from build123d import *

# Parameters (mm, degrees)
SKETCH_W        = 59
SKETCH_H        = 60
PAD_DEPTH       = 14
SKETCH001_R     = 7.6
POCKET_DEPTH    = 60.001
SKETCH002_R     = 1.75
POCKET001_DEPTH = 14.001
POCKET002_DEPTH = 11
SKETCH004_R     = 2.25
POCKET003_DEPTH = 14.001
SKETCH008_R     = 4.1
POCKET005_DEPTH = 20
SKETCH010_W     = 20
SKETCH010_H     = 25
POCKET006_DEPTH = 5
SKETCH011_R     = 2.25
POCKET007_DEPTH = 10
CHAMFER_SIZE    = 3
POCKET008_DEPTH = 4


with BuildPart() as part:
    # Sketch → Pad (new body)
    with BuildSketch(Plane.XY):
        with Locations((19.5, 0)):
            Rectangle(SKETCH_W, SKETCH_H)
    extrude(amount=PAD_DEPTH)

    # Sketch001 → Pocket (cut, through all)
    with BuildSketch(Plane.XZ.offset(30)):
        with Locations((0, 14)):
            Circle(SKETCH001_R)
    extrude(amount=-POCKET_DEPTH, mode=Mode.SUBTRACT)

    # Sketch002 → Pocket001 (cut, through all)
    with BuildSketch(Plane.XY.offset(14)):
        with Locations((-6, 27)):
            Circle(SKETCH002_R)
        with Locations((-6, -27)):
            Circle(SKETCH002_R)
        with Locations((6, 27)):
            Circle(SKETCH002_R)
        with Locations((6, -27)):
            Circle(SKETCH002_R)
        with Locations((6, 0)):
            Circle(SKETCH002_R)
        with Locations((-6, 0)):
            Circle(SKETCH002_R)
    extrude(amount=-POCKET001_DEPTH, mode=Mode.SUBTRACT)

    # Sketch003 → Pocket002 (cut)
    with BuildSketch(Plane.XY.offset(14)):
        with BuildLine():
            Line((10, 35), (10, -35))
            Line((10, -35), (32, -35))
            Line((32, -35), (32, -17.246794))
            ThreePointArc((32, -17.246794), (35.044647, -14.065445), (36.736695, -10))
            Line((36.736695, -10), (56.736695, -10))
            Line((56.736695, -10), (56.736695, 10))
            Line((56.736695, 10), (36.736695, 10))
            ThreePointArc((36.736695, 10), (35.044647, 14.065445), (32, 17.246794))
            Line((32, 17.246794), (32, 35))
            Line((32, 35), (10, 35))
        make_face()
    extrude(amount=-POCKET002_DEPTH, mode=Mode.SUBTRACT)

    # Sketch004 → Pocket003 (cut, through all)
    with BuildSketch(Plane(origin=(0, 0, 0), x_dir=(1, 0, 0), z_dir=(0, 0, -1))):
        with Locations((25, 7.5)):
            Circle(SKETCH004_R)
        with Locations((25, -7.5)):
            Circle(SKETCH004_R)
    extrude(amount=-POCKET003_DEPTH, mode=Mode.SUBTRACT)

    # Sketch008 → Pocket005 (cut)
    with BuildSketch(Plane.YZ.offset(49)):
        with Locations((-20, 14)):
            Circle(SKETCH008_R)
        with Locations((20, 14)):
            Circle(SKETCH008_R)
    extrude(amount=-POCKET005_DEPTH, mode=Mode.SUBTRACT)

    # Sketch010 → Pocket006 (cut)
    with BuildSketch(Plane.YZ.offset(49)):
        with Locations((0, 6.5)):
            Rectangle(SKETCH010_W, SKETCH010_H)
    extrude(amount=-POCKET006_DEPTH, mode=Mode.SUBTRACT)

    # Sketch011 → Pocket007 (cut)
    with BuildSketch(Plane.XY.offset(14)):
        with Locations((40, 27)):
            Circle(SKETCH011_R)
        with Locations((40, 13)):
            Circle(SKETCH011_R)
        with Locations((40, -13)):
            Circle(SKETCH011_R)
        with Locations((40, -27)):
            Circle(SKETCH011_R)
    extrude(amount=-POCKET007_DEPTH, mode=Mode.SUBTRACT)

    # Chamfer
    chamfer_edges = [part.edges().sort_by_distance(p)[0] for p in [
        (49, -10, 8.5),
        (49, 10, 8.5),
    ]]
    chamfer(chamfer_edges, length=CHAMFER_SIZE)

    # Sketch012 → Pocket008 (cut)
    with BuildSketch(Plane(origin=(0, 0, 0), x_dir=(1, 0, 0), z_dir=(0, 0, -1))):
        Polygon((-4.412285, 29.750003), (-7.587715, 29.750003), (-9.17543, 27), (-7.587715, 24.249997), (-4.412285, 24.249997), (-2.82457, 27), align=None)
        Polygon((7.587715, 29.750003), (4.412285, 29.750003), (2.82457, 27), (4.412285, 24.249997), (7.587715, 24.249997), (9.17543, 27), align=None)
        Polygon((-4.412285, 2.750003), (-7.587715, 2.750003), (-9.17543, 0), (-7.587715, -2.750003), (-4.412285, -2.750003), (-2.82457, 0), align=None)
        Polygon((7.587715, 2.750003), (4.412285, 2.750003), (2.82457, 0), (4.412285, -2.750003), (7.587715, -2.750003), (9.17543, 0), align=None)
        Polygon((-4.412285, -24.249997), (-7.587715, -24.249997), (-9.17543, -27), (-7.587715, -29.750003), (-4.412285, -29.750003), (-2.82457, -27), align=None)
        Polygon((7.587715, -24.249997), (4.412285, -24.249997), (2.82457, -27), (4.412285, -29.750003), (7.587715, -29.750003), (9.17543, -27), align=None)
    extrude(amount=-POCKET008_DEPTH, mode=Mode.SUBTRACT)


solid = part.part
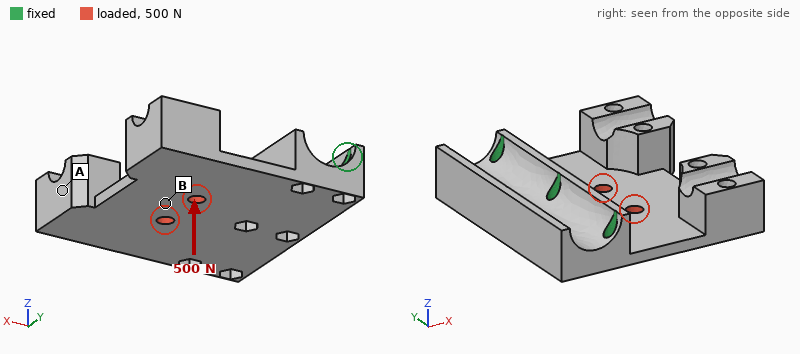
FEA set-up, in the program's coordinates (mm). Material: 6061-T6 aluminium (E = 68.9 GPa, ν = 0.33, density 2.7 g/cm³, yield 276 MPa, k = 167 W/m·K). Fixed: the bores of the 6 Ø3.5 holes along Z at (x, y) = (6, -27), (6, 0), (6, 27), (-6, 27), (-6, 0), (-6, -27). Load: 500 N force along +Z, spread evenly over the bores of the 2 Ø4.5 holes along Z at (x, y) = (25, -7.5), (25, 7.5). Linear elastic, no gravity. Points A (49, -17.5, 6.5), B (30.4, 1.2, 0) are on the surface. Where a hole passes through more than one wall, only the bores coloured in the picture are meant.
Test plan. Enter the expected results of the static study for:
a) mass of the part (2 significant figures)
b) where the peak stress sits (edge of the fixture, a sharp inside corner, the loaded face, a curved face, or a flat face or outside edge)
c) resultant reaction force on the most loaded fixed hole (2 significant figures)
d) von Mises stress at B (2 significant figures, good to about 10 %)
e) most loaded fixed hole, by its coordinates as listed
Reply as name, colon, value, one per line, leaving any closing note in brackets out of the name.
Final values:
mass of the part: 60 g
where the peak stress sits: a flat face or outside edge
resultant reaction force on the most loaded fixed hole: 690 N
von Mises stress at B: 14 MPa
most loaded fixed hole, by its coordinates as listed: (6, 0)
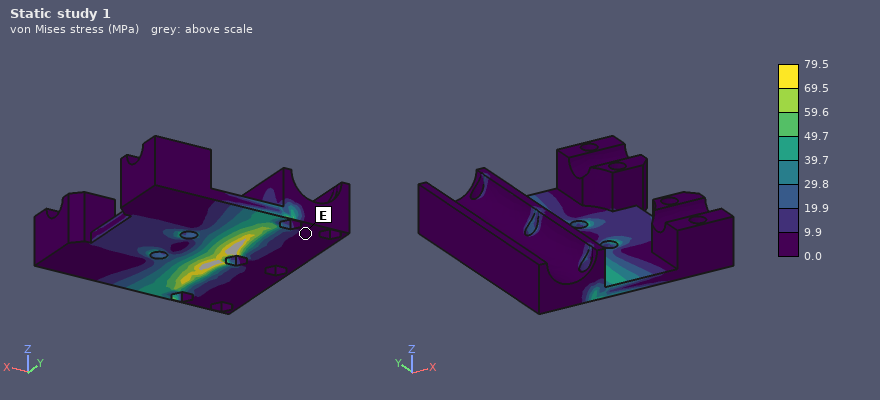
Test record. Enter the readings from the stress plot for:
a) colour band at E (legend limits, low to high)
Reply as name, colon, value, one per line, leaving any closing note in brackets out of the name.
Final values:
colour band at E: 0.0 to 9.9 MPa
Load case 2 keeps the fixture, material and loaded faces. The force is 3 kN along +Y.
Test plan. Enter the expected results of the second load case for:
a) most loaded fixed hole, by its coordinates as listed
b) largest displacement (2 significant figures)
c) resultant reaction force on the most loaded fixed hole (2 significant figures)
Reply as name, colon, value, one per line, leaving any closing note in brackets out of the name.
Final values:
most loaded fixed hole, by its coordinates as listed: (6, 0)
largest displacement: 43 µm
resultant reaction force on the most loaded fixed hole: 1.3 kN
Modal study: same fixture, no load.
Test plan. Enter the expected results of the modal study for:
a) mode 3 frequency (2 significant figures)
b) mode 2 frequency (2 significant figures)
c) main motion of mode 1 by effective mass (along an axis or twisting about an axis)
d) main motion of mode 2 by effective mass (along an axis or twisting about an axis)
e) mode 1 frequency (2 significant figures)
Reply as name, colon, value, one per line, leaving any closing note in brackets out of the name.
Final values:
mode 3 frequency: 3900 Hz
mode 2 frequency: 1500 Hz
main motion of mode 1 by effective mass: along Z
main motion of mode 2 by effective mass: twisting about X
mode 1 frequency: 920 Hz
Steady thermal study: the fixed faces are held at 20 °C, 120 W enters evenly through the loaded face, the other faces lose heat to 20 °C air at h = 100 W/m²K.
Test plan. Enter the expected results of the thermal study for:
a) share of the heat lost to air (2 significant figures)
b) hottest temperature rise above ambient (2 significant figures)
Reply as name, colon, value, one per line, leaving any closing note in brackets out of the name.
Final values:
share of the heat lost to air: 29 %
hottest temperature rise above ambient: 89 K
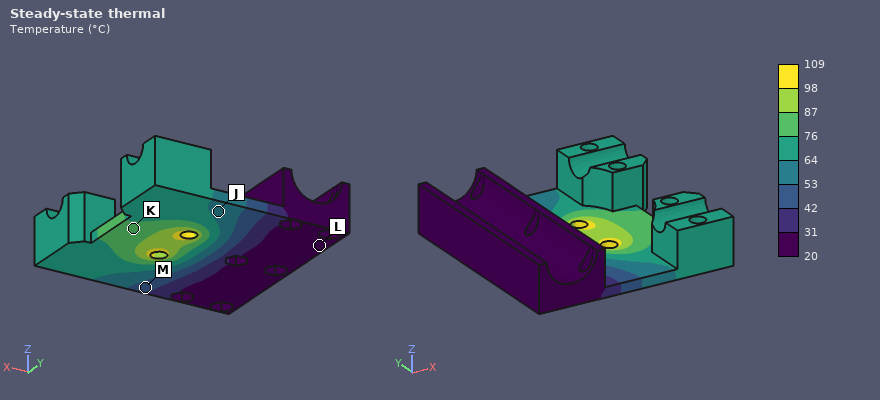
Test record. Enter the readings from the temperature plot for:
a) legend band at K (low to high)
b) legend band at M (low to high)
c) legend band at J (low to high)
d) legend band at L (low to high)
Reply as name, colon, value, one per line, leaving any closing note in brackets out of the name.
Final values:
legend band at K: 76 to 87 °C
legend band at M: 42 to 53 °C
legend band at J: 53 to 64 °C
legend band at L: 20 to 31 °C
